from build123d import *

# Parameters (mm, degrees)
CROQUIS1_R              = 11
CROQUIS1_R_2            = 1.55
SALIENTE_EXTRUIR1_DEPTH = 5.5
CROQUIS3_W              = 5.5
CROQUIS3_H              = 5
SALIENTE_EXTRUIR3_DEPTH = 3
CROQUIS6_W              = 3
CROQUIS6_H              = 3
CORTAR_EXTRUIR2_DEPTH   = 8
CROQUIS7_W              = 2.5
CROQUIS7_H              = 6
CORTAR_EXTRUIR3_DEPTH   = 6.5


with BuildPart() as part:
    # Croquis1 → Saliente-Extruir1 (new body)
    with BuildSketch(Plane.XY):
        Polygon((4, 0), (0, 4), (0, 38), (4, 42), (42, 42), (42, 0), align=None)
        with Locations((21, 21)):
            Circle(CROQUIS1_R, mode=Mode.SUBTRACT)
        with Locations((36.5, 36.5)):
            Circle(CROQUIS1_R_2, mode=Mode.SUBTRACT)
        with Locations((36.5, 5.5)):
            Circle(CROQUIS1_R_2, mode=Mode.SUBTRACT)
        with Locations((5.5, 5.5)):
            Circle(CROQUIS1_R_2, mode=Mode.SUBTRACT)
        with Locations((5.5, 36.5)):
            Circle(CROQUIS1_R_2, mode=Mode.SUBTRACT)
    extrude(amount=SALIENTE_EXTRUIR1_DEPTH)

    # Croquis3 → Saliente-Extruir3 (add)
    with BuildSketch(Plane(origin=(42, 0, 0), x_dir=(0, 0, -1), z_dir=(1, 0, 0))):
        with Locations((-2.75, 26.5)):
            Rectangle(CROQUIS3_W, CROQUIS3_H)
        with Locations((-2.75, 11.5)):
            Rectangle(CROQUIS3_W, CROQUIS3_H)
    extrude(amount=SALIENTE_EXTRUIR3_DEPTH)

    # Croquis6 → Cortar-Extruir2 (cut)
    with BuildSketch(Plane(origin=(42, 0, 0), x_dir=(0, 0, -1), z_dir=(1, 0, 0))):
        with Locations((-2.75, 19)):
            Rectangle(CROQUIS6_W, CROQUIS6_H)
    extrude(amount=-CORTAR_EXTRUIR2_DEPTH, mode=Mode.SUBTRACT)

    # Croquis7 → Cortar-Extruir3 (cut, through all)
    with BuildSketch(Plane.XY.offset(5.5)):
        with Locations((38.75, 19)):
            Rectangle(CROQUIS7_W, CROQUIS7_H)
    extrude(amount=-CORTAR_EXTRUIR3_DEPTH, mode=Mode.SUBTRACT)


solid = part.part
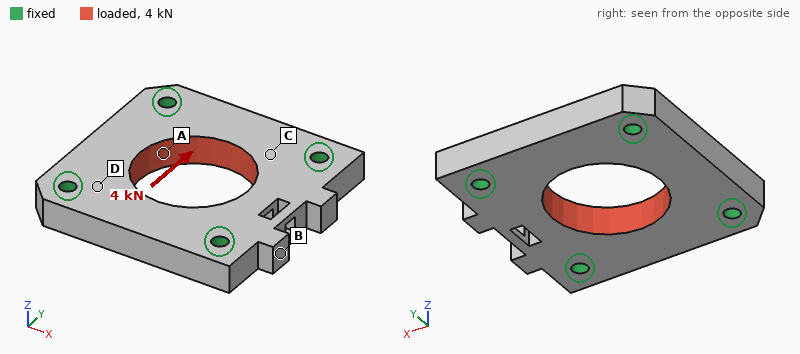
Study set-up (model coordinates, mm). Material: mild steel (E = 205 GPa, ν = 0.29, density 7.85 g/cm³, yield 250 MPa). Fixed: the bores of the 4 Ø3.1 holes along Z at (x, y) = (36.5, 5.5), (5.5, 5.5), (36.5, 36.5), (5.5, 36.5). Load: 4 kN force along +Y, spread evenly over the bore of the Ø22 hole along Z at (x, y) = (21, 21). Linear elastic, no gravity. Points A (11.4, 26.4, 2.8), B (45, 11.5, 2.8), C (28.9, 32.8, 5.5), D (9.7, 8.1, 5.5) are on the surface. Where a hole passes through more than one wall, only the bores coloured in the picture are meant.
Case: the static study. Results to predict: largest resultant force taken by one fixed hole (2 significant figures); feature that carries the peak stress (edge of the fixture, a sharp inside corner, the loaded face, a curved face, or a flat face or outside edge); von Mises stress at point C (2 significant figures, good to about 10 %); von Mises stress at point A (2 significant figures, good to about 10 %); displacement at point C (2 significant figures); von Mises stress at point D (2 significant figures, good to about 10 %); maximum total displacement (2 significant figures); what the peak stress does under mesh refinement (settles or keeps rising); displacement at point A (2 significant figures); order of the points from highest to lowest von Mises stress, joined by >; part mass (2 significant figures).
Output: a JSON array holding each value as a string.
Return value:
["1.1 kN", "edge of the fixture", "13 MPa", "25 MPa", "1.4 µm", "17 MPa", "2.4 µm", "keeps rising", "1.2 µm", "A > D > C > B", "58 g"]
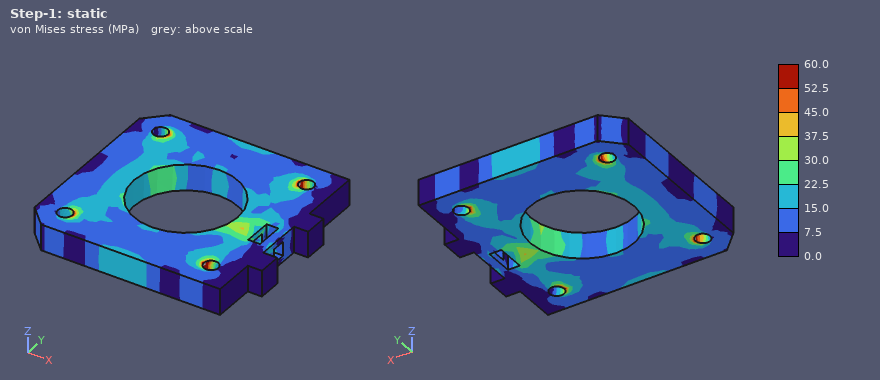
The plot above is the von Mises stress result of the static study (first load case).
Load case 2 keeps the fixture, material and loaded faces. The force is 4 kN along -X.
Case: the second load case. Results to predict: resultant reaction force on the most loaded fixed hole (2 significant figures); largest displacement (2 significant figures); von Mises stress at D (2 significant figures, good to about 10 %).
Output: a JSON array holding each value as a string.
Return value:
["1.1 kN", "2.7 µm", "18 MPa"]
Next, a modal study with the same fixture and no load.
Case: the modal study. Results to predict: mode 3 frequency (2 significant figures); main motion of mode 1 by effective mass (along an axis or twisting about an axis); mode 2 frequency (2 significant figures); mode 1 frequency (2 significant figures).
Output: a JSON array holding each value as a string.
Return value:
["26 kHz", "along Z", "25 kHz", "24 kHz"]
